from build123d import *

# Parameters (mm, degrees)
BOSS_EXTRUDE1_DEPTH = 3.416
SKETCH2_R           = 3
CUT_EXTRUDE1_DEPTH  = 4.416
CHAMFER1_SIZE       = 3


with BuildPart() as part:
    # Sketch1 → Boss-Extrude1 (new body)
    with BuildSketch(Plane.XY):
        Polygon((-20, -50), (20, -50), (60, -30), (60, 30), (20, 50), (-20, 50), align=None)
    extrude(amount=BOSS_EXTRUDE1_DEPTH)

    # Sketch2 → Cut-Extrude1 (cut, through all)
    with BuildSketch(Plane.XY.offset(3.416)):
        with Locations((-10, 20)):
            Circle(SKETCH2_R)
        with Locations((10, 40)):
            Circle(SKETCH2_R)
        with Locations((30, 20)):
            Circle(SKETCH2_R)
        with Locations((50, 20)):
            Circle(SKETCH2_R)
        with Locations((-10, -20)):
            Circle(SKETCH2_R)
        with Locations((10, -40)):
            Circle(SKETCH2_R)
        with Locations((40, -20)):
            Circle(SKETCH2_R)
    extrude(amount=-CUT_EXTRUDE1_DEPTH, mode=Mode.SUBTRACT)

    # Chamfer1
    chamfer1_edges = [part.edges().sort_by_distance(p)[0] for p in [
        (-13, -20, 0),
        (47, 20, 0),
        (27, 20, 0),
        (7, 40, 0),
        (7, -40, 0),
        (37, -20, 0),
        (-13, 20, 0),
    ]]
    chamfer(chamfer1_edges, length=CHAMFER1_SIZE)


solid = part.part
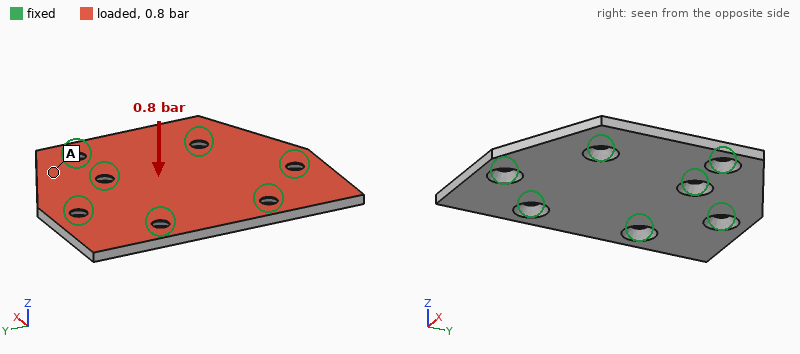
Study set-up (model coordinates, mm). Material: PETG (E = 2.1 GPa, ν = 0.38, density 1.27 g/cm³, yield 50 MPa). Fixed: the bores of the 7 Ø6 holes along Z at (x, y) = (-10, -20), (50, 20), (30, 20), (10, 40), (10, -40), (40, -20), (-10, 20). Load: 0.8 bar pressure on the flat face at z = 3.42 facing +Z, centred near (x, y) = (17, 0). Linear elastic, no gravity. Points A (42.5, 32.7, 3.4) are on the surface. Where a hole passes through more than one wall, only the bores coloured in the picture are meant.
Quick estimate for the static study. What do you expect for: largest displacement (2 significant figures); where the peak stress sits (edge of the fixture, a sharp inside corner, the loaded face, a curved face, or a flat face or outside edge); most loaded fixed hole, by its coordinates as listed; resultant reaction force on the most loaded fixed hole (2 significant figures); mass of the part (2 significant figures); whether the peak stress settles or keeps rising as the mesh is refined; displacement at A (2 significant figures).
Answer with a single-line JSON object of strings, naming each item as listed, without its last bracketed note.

{"largest displacement": "0.51 mm", "where the peak stress sits": "edge of the fixture", "most loaded fixed hole, by its coordinates as listed": "(40, -20)", "resultant reaction force on the most loaded fixed hole": "120 N", "mass of the part": "29 g", "whether the peak stress settles or keeps rising as the mesh is refined": "keeps rising", "displacement at A": "0.080 mm"}
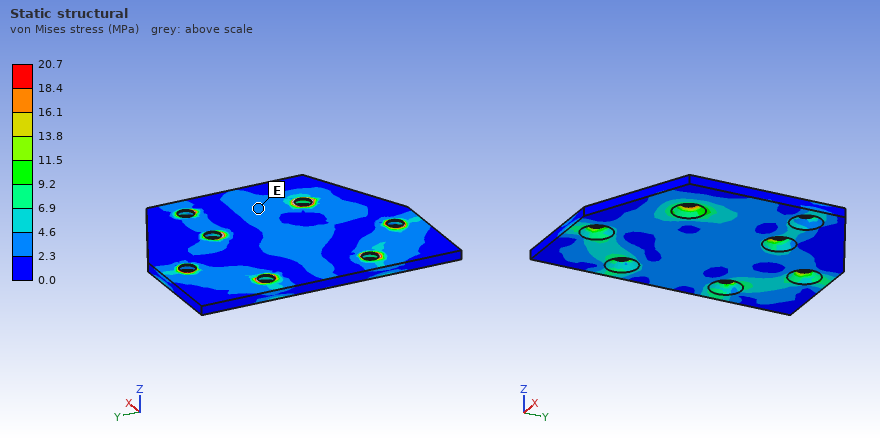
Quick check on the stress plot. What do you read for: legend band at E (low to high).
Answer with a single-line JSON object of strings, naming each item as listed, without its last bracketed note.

{"legend band at E": "2.3 to 4.6 MPa"}
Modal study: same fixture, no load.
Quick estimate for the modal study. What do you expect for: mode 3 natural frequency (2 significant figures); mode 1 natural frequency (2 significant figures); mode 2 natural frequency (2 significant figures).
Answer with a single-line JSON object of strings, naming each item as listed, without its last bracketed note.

{"mode 3 natural frequency": "1400 Hz", "mode 1 natural frequency": "1200 Hz", "mode 2 natural frequency": "1200 Hz"}
